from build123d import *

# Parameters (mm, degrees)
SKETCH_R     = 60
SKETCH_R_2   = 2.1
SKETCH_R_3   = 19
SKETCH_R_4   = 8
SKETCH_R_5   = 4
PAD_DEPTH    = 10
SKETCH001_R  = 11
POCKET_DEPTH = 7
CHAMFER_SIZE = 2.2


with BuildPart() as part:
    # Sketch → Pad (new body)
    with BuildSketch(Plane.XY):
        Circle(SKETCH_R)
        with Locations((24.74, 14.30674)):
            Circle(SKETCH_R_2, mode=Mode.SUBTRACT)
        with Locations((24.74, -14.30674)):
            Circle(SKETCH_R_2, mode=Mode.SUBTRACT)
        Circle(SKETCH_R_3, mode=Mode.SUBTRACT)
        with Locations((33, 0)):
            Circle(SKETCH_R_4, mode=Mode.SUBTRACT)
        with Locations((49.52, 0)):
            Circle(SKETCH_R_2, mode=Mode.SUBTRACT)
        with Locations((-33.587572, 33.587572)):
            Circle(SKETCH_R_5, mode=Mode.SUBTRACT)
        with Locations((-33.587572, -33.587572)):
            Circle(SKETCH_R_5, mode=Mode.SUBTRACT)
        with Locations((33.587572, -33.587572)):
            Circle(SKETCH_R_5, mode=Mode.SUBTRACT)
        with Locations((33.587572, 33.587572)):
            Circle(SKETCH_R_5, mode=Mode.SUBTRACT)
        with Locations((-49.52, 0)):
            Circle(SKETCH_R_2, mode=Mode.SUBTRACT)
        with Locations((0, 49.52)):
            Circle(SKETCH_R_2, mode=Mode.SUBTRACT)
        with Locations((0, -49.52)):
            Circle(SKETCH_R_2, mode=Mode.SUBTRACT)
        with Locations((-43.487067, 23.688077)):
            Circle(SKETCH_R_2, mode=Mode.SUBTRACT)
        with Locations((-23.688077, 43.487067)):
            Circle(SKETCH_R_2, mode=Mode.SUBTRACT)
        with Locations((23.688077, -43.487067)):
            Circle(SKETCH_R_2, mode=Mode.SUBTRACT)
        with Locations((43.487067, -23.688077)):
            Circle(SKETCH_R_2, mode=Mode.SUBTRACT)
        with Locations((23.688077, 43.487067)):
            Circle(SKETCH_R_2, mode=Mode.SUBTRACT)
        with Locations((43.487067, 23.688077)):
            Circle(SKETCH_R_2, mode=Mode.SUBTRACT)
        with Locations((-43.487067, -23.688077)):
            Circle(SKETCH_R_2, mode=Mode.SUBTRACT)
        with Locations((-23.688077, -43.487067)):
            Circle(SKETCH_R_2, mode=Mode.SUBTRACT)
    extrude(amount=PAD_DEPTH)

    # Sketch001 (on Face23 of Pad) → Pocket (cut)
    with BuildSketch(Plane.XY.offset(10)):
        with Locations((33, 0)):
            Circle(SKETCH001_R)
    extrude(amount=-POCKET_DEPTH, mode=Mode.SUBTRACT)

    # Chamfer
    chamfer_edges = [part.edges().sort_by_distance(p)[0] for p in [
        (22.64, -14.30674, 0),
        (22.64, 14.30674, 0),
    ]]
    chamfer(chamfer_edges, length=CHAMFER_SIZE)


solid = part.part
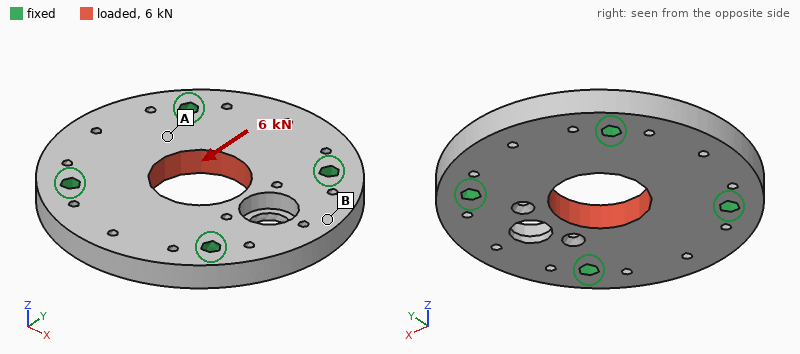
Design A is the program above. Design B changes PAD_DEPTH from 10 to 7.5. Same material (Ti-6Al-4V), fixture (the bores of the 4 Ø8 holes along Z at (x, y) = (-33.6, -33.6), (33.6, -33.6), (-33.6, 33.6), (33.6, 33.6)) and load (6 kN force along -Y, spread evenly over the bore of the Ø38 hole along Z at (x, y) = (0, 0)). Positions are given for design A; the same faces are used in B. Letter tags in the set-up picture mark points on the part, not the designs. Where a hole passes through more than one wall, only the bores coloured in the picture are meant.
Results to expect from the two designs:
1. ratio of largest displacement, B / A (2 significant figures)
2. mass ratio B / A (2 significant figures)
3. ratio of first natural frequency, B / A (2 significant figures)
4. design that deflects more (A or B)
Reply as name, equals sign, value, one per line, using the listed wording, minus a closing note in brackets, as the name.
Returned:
ratio of largest displacement, B / A = 1.3
mass ratio B / A = 0.75
ratio of first natural frequency, B / A = 0.80
design that deflects more = B
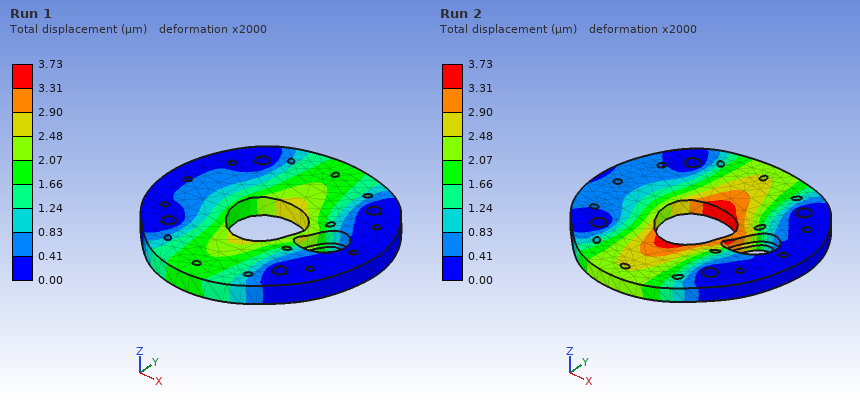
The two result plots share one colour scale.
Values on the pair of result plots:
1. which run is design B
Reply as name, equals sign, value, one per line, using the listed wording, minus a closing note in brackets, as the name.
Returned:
which run is design B = Run 2
